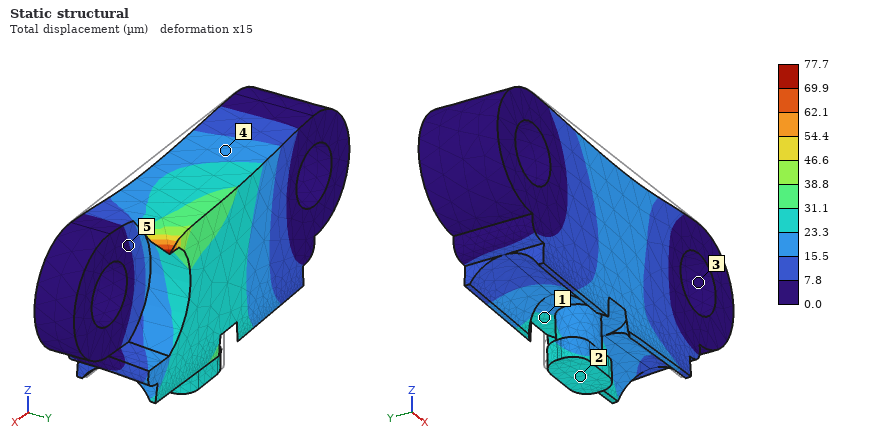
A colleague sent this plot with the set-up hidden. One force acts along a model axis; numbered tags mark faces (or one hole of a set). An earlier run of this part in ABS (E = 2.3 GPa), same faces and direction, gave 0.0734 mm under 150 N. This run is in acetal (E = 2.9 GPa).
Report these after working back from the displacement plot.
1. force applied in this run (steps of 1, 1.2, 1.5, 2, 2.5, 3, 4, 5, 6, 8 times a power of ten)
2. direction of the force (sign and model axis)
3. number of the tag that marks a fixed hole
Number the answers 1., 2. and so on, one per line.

1. 200 N
2. -Z
3. 3
